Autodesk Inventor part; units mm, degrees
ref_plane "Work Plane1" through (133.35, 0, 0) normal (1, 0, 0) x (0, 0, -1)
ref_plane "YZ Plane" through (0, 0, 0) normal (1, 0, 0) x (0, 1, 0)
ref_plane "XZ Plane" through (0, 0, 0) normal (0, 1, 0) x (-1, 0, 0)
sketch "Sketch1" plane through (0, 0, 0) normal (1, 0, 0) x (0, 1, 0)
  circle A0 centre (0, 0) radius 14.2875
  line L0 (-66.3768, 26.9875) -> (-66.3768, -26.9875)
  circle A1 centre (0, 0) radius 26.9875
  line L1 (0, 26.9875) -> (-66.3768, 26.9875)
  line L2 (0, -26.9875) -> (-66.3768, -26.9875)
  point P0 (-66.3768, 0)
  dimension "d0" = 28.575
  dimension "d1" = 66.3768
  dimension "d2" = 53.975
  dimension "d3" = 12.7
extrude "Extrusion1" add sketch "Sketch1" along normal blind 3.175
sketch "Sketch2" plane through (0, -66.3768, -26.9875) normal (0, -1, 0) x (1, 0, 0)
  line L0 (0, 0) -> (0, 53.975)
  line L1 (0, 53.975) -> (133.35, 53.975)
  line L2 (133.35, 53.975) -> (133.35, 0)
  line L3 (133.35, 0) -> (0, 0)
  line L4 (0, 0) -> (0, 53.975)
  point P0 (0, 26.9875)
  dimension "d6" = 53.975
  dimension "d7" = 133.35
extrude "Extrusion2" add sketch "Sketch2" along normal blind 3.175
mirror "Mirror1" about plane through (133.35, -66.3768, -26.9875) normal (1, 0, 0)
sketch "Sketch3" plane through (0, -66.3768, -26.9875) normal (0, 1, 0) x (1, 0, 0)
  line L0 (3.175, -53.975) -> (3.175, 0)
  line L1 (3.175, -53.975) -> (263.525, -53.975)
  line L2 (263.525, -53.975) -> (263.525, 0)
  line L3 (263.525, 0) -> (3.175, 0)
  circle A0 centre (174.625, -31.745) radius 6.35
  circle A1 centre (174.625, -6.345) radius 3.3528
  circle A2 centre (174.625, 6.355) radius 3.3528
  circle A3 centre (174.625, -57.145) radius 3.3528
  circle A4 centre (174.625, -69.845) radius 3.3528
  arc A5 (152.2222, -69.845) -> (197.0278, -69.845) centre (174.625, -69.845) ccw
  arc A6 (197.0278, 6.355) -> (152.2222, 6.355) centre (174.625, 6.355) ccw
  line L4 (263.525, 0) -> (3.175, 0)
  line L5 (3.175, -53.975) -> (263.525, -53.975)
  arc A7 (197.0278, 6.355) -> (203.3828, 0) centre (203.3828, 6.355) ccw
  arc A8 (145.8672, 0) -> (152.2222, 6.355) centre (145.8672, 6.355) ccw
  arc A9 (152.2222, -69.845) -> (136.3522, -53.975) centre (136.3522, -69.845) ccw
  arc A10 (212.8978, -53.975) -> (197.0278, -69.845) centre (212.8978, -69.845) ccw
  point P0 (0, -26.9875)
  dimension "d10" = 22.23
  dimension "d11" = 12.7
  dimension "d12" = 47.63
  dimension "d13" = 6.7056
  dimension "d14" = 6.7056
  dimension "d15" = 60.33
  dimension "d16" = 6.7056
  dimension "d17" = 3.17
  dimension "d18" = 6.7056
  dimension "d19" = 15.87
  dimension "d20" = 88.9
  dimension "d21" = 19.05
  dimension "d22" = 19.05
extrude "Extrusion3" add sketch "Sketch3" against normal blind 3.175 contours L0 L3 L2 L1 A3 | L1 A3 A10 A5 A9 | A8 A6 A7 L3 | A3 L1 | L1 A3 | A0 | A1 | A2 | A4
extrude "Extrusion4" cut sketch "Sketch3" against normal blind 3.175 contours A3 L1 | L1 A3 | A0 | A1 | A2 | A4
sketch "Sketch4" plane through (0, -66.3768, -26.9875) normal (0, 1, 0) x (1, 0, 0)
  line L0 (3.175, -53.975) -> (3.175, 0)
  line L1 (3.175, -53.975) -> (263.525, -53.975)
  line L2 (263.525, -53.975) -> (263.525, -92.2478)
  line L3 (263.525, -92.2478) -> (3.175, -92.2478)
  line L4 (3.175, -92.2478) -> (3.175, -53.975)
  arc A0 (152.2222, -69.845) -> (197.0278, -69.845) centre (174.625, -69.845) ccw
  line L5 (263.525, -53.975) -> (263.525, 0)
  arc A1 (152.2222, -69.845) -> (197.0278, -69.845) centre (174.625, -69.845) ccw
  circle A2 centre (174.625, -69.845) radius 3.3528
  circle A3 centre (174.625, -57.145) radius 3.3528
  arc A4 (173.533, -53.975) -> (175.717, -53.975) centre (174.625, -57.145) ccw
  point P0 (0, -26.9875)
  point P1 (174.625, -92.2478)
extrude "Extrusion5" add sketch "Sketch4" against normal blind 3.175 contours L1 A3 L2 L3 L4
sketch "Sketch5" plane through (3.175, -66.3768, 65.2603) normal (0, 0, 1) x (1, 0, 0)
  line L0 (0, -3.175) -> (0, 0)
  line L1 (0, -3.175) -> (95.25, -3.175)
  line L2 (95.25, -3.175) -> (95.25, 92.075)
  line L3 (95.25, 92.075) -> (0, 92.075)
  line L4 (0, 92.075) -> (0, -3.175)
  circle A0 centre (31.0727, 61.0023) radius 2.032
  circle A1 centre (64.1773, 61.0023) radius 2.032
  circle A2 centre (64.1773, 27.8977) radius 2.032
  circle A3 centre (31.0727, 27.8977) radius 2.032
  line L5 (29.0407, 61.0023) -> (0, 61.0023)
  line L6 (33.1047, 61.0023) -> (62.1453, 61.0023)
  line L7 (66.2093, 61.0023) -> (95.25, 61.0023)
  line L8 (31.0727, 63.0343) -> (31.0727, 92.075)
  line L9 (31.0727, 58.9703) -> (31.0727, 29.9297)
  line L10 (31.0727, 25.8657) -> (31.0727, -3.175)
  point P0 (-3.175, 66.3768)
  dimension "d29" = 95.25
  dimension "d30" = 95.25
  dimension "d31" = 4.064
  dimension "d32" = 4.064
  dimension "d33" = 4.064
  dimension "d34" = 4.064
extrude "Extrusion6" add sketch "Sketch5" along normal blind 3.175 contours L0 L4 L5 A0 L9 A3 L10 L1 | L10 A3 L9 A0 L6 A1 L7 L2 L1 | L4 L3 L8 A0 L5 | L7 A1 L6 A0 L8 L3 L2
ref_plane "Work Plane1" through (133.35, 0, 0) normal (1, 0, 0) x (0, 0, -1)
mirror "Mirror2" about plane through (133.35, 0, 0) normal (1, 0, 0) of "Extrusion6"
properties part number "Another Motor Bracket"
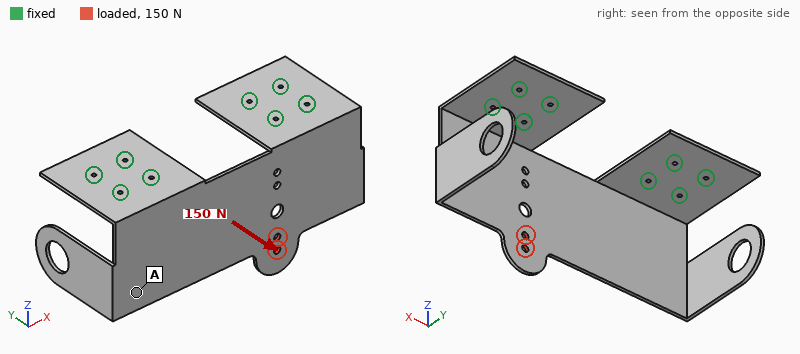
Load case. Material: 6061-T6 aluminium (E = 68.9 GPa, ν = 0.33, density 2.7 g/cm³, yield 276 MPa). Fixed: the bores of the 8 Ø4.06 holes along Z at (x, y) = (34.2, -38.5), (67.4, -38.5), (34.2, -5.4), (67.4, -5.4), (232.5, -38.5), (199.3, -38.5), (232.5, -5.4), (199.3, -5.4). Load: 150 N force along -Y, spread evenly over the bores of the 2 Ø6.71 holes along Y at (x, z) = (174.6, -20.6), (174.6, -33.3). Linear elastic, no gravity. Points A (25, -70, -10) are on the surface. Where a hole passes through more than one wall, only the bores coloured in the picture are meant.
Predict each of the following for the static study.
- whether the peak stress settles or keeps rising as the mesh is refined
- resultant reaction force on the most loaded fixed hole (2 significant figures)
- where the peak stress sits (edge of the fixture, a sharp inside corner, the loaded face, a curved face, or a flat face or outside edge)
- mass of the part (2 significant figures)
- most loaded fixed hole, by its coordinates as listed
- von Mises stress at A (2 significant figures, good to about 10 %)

keeps rising
120 N
edge of the fixture
440 g
(232.5, -38.5)
12 MPa
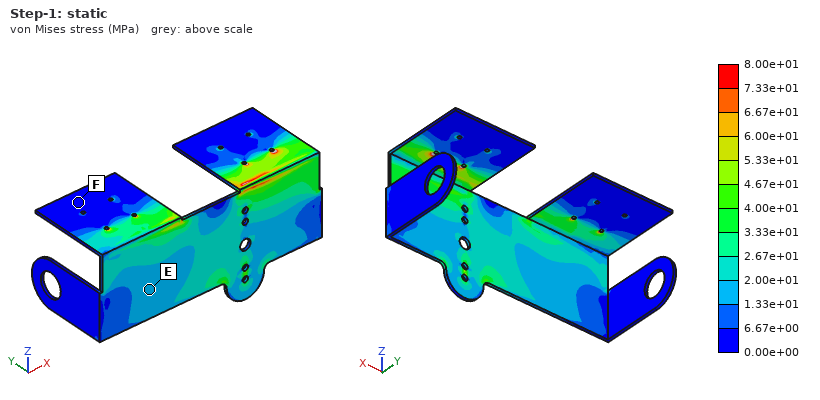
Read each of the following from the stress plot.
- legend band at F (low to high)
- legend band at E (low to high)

0.00e+00 to 6.67e+00 MPa
1.33e+01 to 2.00e+01 MPa
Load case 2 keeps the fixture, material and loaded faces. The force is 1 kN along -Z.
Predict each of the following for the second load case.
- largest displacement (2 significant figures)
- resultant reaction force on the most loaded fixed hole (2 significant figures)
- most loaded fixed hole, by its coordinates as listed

1.9 mm
550 N
(232.5, -38.5)
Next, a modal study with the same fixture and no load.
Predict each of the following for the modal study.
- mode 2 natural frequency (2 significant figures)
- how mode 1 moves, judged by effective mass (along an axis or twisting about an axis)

150 Hz
along Y
